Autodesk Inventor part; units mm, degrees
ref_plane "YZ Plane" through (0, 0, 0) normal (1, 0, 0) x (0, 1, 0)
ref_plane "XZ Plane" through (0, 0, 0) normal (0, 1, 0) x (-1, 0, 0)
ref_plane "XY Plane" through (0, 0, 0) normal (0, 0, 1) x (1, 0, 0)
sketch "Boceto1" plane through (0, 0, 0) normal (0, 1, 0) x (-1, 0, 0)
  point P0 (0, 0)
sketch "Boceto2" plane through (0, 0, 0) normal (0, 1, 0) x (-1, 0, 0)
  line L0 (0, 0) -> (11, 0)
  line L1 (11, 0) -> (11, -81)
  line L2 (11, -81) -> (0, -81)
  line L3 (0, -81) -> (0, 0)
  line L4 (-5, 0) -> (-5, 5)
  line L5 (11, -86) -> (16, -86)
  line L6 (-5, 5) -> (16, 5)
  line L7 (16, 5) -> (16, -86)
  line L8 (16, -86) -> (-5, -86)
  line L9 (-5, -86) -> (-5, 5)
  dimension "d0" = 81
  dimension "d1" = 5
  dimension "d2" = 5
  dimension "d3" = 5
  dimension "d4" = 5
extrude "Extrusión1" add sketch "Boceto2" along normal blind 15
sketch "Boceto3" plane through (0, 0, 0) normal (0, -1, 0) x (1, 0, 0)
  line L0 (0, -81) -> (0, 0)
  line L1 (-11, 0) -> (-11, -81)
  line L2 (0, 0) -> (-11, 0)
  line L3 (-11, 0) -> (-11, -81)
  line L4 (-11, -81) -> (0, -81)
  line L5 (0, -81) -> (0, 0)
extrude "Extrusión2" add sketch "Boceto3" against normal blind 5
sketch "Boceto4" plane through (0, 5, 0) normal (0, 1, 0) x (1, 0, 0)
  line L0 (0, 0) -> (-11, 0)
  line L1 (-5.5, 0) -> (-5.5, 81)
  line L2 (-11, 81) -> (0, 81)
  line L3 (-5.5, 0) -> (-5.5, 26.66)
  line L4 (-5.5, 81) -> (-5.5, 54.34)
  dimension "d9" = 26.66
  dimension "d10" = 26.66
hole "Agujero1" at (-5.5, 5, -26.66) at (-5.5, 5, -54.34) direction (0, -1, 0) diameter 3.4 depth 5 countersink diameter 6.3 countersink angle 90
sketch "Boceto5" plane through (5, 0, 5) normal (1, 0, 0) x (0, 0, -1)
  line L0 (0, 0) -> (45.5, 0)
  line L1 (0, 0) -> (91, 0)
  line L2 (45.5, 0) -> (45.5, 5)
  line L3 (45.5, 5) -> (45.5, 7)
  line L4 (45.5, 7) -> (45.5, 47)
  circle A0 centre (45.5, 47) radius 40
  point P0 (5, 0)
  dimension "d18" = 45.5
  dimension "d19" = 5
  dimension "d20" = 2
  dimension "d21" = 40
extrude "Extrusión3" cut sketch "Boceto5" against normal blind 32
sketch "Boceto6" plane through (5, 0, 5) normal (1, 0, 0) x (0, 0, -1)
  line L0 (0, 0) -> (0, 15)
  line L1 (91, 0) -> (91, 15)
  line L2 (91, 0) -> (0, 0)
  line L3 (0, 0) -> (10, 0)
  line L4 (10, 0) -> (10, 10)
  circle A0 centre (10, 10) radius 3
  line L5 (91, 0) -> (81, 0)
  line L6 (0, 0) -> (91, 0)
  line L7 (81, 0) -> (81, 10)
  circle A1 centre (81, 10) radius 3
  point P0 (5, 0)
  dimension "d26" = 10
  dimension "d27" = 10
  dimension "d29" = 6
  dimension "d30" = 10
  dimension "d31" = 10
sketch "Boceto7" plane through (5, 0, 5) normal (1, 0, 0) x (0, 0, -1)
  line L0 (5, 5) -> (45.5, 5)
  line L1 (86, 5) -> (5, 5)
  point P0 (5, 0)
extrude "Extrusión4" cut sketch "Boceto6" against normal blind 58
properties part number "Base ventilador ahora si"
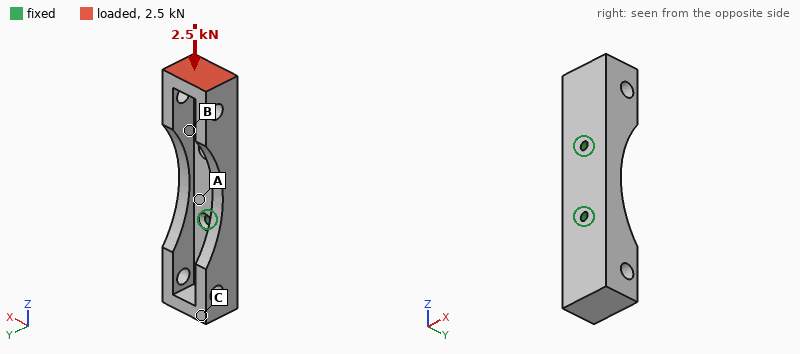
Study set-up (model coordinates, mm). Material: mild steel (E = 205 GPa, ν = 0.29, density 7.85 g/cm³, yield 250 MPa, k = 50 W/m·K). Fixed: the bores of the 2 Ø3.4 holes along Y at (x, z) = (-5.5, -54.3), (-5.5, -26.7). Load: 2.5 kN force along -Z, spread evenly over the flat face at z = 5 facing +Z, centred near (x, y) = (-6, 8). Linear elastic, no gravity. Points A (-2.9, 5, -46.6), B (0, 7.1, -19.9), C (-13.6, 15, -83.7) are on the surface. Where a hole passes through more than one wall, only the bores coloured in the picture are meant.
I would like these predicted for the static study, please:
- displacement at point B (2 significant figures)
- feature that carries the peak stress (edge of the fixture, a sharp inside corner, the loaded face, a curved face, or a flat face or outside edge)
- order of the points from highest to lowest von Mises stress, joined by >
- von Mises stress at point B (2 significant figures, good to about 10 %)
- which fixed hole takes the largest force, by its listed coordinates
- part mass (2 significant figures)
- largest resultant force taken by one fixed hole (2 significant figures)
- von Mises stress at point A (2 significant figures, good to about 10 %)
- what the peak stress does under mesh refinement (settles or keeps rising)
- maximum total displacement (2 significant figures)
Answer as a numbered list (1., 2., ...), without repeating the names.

1. 6.8 µm
2. edge of the fixture
3. B > A > C
4. 24 MPa
5. (-5.5, -26.7)
6. 130 g
7. 1.5 kN
8. 18 MPa
9. keeps rising
10. 33 µm
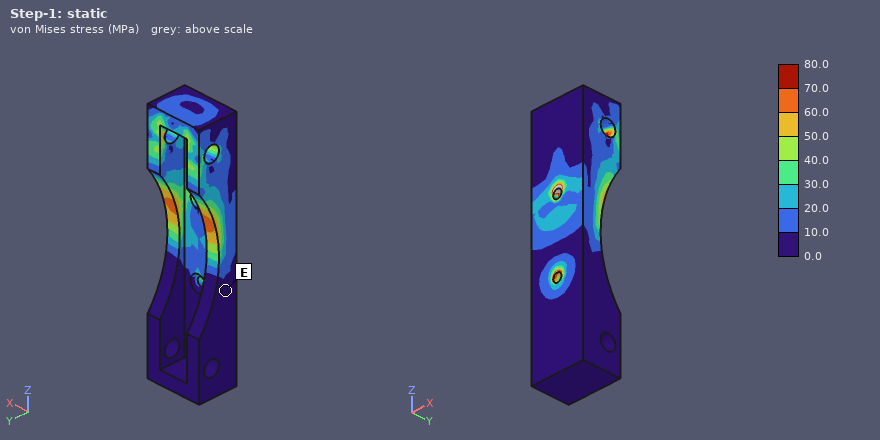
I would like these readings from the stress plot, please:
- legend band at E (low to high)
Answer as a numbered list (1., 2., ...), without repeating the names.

1. 0.0 to 10.0 MPa
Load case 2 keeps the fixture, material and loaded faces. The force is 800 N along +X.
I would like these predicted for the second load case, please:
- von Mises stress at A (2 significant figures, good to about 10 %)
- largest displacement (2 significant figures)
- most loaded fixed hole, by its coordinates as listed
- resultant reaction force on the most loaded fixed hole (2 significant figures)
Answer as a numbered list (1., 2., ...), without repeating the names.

1. 11 MPa
2. 33 µm
3. (-5.5, -26.7)
4. 1.6 kN
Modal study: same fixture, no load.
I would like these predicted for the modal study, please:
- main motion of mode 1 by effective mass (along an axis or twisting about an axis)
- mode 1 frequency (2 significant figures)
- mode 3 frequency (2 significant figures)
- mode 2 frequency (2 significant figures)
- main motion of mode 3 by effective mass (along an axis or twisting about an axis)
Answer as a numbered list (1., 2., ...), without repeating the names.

1. along Y
2. 3800 Hz
3. 5200 Hz
4. 4100 Hz
5. along X
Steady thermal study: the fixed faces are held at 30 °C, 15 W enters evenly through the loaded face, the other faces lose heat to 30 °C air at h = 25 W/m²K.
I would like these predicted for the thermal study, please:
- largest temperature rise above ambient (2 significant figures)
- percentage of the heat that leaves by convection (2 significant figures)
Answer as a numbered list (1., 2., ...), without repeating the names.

1. 59 K
2. 18 %
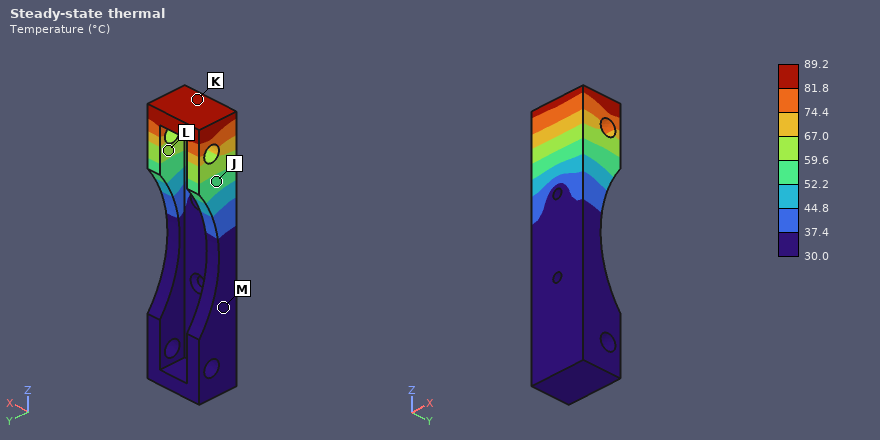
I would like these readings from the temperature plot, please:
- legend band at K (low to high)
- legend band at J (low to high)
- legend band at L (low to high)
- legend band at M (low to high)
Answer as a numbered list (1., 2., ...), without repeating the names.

1. 81.8 to 89.2 °C
2. 52.2 to 59.6 °C
3. 59.6 to 67.0 °C
4. 30.0 to 37.4 °C
